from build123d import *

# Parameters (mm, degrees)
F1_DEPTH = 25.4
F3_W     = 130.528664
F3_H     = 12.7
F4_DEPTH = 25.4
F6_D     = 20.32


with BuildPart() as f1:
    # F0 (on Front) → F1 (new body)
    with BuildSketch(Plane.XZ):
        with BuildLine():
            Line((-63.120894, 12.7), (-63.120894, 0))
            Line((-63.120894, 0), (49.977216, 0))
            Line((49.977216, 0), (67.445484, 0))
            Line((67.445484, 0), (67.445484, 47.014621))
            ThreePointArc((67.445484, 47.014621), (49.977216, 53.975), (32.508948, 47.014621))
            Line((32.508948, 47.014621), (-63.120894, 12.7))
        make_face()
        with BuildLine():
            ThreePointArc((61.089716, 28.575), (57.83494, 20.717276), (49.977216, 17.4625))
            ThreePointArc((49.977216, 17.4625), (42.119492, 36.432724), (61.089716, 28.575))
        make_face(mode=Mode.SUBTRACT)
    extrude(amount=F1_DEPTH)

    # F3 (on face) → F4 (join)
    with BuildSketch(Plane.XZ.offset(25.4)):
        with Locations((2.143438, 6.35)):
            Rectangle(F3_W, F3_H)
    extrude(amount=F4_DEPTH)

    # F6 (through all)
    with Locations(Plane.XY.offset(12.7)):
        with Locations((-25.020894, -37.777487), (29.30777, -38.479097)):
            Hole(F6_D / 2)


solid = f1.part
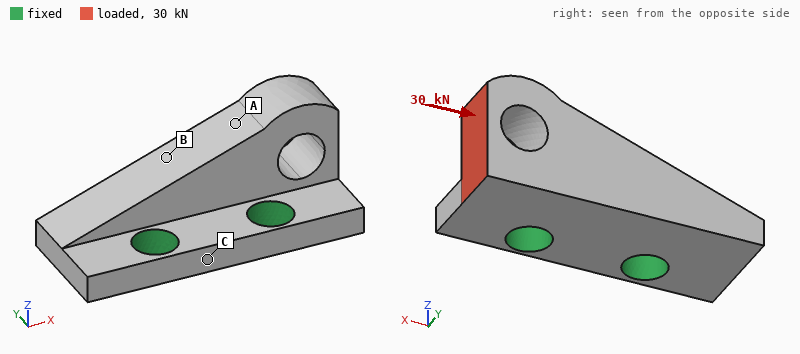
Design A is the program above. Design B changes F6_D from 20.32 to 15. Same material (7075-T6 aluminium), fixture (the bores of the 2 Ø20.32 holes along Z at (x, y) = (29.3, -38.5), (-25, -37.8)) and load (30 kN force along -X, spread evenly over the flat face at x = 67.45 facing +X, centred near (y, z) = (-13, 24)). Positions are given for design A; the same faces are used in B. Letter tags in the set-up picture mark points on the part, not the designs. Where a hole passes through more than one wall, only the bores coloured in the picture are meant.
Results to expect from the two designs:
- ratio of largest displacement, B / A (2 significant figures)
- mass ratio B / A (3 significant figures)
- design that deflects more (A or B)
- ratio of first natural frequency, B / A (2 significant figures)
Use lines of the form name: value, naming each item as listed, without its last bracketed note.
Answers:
ratio of largest displacement, B / A: 1.2
mass ratio B / A: 1.03
design that deflects more: B
ratio of first natural frequency, B / A: 0.87
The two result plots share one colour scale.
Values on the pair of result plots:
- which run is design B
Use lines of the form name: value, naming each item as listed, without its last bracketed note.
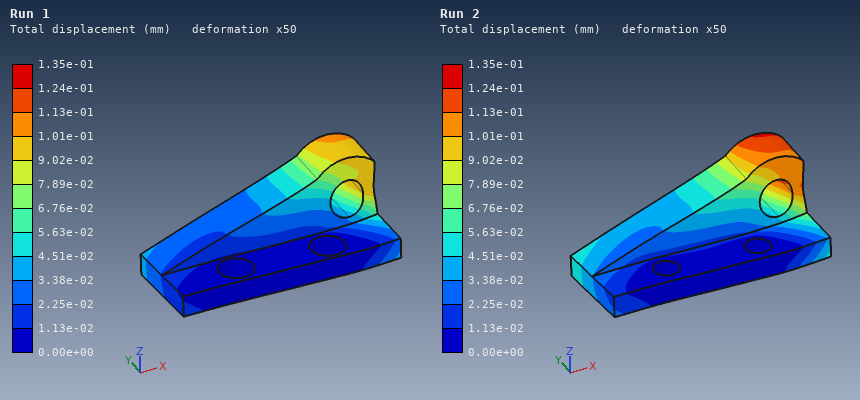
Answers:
which run is design B: Run 2
